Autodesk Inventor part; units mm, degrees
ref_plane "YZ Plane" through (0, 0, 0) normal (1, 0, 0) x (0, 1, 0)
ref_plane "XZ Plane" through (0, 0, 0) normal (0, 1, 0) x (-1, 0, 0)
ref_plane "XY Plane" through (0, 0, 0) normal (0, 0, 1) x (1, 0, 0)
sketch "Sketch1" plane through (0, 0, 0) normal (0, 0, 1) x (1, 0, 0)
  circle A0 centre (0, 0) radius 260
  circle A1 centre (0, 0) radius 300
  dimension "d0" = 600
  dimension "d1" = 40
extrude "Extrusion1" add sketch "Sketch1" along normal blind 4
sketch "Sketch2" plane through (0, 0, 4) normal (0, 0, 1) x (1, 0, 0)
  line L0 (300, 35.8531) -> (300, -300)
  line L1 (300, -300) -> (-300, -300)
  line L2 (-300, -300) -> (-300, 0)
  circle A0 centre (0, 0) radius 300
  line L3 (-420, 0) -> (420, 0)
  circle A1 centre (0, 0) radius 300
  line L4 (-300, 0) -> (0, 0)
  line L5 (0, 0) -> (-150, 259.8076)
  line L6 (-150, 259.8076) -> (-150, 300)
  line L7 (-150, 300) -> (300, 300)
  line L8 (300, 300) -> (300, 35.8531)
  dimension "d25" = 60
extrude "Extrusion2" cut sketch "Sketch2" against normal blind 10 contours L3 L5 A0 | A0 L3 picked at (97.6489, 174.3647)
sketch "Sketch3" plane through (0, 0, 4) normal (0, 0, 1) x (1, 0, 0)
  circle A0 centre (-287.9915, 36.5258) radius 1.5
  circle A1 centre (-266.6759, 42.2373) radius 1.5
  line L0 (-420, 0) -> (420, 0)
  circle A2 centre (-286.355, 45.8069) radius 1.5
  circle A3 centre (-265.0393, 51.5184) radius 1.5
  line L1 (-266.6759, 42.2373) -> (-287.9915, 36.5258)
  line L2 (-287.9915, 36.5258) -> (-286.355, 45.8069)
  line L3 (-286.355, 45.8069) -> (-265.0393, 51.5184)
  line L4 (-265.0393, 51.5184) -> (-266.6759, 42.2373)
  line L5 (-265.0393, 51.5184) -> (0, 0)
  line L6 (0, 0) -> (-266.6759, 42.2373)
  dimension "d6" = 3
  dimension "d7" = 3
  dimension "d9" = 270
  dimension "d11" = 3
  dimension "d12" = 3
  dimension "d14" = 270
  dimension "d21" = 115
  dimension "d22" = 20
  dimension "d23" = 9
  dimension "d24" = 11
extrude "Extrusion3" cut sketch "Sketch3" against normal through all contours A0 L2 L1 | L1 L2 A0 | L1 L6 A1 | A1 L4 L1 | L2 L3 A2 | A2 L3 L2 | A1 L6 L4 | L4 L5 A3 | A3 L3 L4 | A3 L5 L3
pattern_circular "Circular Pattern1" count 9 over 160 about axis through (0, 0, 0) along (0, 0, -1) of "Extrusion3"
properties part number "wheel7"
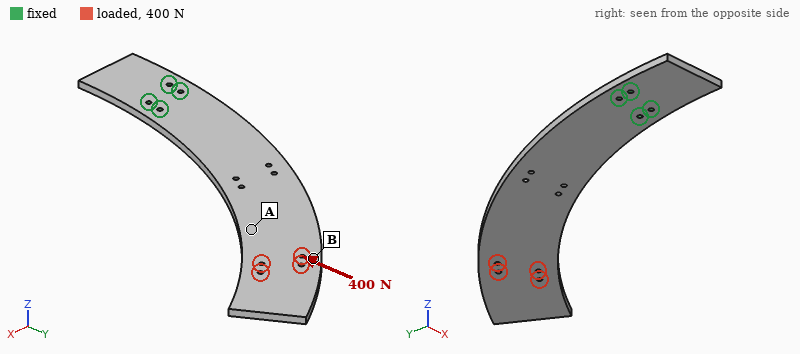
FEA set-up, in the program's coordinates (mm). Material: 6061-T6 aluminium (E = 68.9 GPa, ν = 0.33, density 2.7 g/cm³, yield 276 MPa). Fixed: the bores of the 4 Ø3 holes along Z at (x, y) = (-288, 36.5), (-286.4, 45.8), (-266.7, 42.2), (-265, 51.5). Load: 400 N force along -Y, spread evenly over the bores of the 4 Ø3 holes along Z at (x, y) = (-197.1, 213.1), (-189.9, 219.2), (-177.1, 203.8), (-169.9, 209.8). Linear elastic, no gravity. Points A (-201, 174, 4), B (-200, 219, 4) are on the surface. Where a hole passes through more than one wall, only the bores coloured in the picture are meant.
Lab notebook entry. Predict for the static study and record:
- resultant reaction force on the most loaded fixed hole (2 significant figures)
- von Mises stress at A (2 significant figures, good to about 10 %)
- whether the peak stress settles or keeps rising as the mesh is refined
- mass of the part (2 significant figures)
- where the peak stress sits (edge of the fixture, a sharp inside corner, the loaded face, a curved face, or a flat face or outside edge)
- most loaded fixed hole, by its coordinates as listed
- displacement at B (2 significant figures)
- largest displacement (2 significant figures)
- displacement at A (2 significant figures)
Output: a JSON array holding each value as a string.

["1.3 kN", "9.4 MPa", "keeps rising", "130 g", "edge of the fixture", "(-265, 51.5)", "0.37 mm", "0.56 mm", "0.26 mm"]
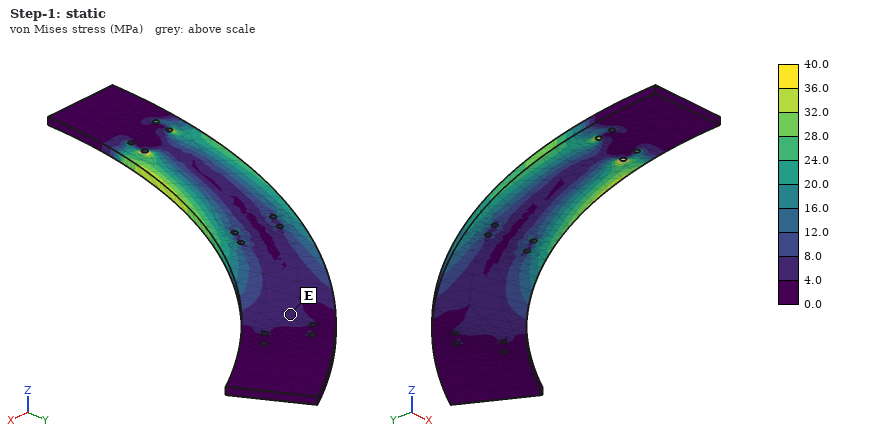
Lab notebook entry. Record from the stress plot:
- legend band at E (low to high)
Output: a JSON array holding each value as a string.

["4.0 to 8.0 MPa"]
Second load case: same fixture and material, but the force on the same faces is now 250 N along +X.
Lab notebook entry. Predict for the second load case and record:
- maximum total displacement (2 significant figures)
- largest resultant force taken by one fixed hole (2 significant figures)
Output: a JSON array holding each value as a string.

["0.51 mm", "1.3 kN"]
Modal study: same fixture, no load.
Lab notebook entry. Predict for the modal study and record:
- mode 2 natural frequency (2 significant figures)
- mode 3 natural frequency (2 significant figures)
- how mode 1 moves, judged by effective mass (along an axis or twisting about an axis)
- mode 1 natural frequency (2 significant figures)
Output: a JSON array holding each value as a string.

["320 Hz", "520 Hz", "along Z", "58 Hz"]
